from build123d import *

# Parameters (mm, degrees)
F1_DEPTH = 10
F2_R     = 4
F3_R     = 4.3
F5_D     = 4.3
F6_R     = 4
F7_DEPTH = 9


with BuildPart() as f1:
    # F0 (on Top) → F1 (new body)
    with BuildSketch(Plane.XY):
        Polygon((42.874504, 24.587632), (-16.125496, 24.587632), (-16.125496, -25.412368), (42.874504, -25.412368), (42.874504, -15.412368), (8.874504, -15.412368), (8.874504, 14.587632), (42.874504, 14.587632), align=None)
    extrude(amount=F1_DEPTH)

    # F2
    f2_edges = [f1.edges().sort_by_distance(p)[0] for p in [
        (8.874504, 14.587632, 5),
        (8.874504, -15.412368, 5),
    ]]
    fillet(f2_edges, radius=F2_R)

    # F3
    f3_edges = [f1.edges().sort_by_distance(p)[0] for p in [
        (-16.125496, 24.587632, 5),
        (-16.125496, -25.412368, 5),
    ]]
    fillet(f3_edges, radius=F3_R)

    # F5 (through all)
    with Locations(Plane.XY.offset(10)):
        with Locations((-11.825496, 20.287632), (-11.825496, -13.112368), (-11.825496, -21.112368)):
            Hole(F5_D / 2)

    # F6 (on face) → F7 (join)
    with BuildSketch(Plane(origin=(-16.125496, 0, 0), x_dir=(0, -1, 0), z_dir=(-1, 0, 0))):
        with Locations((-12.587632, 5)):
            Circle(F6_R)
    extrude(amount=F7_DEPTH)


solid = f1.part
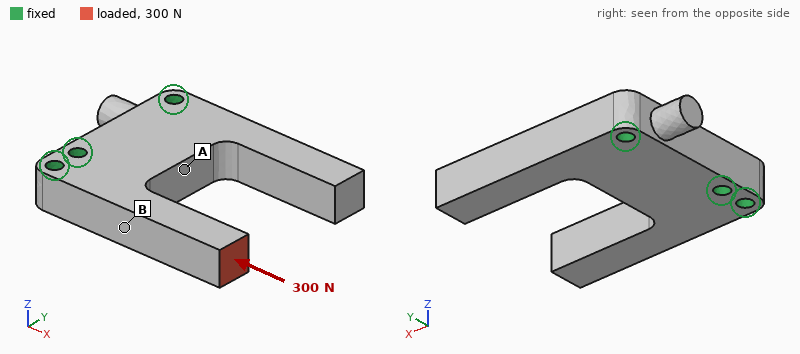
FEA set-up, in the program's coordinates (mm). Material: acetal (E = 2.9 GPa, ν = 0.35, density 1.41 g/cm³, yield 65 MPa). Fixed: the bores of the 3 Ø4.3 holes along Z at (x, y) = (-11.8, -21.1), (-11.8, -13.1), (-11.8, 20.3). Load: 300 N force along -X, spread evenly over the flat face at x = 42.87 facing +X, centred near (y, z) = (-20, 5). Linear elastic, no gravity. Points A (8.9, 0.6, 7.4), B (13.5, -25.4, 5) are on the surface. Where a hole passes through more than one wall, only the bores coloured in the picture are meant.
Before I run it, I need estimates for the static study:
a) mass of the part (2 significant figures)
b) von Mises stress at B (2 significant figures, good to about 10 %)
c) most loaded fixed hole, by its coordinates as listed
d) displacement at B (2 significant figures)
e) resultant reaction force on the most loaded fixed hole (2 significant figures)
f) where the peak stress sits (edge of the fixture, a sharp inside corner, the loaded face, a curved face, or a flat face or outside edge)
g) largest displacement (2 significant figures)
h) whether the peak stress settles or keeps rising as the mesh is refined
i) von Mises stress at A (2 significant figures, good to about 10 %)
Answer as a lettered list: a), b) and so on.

a) 27 g
b) 3.1 MPa
c) (-11.8, -21.1)
d) 33 µm
e) 200 N
f) edge of the fixture
g) 81 µm
h) keeps rising
i) 0.47 MPa
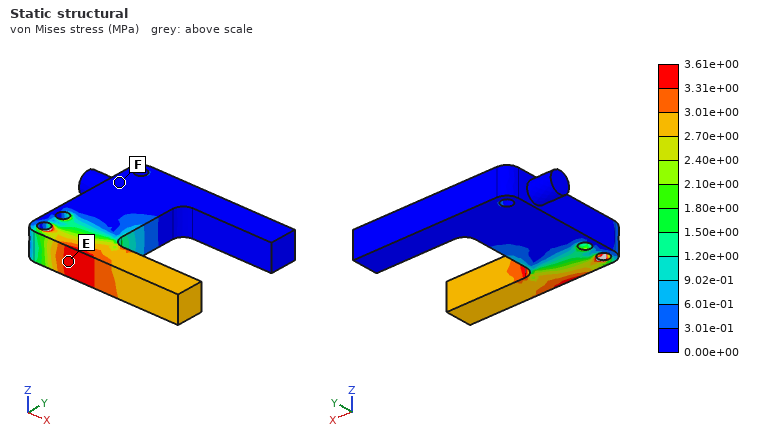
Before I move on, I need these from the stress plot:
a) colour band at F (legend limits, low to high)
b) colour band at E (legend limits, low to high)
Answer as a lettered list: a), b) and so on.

a) 0.00e+00 to 3.01e-01 MPa
b) 3.31e+00 to 3.61e+00 MPa
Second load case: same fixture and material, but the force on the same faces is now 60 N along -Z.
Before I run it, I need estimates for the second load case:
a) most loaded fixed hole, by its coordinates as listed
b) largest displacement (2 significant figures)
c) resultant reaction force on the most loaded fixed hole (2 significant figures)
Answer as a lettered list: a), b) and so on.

a) (-11.8, -13.1)
b) 0.86 mm
c) 50 N
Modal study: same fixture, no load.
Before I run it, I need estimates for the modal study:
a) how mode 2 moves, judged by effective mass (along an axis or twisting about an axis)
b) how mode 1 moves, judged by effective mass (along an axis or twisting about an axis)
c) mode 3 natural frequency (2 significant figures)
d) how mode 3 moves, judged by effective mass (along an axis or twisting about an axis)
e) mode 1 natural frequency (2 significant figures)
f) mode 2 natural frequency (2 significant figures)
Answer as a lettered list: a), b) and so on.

a) twisting about X
b) along Z
c) 1500 Hz
d) along Y
e) 940 Hz
f) 1100 Hz
